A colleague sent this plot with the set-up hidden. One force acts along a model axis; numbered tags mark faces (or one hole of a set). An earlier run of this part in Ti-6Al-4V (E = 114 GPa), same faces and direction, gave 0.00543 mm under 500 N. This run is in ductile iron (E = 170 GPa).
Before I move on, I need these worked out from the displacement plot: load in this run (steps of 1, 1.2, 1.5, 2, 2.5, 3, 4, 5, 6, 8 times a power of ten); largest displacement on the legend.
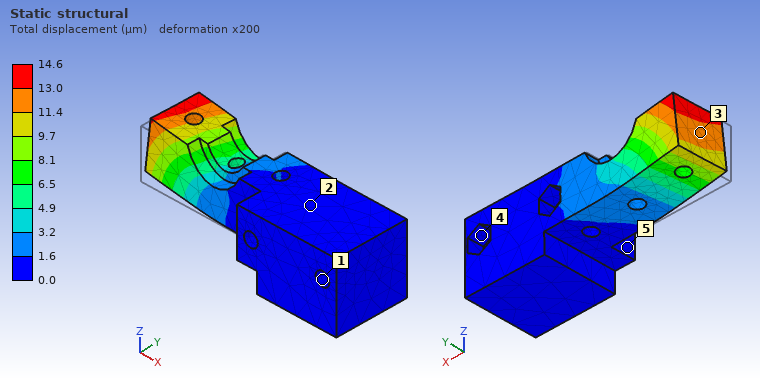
2 kN
14.6 µm
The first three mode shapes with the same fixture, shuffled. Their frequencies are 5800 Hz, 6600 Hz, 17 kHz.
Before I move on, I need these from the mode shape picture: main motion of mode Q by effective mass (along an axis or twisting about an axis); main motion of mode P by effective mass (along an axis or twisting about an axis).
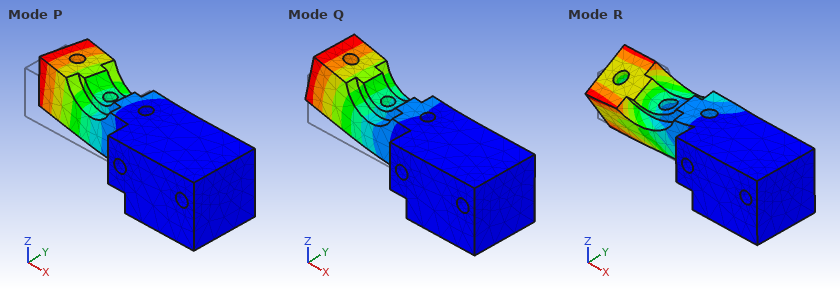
along Z
along Y
